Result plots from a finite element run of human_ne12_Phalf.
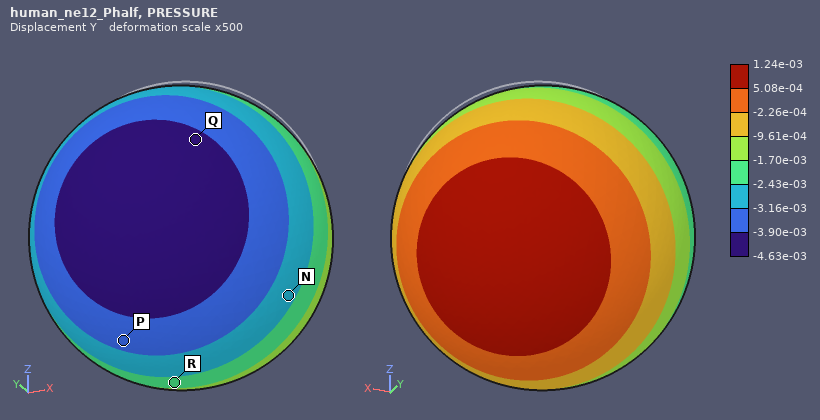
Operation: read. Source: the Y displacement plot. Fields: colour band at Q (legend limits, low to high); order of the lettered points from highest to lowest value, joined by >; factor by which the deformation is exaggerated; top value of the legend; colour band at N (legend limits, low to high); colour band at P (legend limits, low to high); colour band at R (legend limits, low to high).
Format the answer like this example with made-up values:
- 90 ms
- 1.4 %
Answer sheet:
- -4.63e-03 to -3.90e-03
- R > N > P > Q
- 500
- 1.24e-03
- -3.16e-03 to -2.43e-03
- -3.90e-03 to -3.16e-03
- -2.43e-03 to -1.70e-03
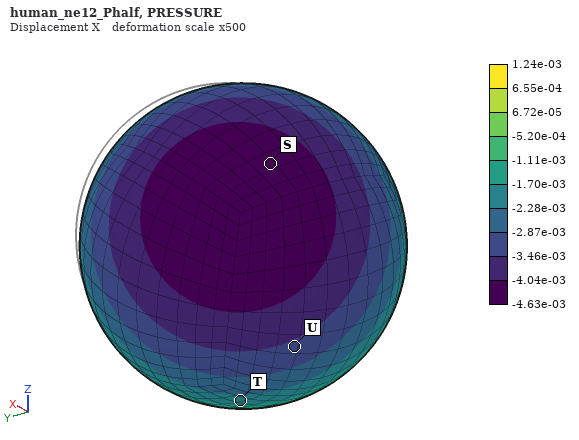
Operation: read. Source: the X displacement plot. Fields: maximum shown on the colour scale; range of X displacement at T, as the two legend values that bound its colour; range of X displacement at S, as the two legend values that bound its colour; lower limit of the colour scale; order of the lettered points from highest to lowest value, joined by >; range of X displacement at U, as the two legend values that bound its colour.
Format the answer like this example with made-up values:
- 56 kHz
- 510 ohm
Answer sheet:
- 1.24e-03
- -2.28e-03 to -1.70e-03
- -4.63e-03 to -4.04e-03
- -4.63e-03
- T > U > S
- -3.46e-03 to -2.87e-03
